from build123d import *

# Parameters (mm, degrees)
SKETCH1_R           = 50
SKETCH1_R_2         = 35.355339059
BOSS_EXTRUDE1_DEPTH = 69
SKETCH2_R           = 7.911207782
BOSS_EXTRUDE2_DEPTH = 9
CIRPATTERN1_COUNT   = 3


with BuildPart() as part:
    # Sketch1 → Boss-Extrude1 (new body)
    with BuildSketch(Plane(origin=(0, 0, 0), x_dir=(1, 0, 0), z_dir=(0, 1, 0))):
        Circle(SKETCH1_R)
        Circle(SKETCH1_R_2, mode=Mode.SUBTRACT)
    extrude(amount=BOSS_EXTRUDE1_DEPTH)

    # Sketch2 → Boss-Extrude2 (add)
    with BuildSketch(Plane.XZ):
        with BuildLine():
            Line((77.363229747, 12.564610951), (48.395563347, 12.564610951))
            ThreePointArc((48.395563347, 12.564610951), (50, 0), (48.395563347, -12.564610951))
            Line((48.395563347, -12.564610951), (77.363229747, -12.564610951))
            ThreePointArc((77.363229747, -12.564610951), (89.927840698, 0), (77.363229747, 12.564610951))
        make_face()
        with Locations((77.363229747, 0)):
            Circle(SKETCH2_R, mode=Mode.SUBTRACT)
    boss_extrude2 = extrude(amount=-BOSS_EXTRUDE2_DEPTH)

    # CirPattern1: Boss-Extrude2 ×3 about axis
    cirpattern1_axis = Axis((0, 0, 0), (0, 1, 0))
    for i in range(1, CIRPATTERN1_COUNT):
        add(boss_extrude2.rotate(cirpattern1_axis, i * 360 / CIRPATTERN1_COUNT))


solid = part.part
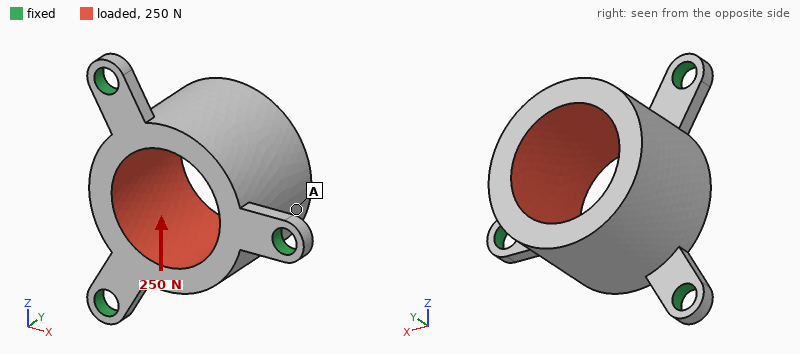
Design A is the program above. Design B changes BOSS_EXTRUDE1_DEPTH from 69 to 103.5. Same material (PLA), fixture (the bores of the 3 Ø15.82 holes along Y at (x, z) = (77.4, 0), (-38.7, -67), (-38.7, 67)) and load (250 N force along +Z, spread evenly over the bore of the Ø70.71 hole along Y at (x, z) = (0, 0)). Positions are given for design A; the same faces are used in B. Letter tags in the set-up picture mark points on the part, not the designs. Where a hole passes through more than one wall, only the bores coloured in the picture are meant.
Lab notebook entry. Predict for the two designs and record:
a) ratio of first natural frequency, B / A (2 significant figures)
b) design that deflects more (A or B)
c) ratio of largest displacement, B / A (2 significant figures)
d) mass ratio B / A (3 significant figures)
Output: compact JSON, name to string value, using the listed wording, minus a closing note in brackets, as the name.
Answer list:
{"ratio of first natural frequency, B / A": "0.62", "design that deflects more": "B", "ratio of largest displacement, B / A": "2.0", "mass ratio B / A": "1.47"}
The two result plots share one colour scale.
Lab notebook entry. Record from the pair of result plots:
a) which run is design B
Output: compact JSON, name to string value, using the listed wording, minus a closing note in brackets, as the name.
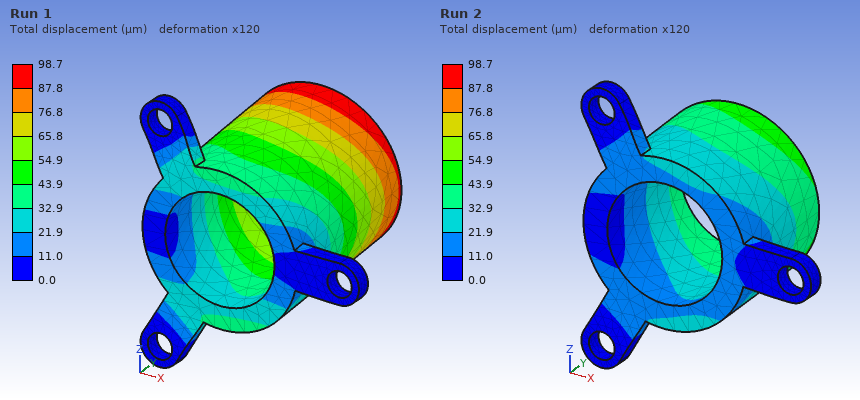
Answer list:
{"which run is design B": "Run 1"}
